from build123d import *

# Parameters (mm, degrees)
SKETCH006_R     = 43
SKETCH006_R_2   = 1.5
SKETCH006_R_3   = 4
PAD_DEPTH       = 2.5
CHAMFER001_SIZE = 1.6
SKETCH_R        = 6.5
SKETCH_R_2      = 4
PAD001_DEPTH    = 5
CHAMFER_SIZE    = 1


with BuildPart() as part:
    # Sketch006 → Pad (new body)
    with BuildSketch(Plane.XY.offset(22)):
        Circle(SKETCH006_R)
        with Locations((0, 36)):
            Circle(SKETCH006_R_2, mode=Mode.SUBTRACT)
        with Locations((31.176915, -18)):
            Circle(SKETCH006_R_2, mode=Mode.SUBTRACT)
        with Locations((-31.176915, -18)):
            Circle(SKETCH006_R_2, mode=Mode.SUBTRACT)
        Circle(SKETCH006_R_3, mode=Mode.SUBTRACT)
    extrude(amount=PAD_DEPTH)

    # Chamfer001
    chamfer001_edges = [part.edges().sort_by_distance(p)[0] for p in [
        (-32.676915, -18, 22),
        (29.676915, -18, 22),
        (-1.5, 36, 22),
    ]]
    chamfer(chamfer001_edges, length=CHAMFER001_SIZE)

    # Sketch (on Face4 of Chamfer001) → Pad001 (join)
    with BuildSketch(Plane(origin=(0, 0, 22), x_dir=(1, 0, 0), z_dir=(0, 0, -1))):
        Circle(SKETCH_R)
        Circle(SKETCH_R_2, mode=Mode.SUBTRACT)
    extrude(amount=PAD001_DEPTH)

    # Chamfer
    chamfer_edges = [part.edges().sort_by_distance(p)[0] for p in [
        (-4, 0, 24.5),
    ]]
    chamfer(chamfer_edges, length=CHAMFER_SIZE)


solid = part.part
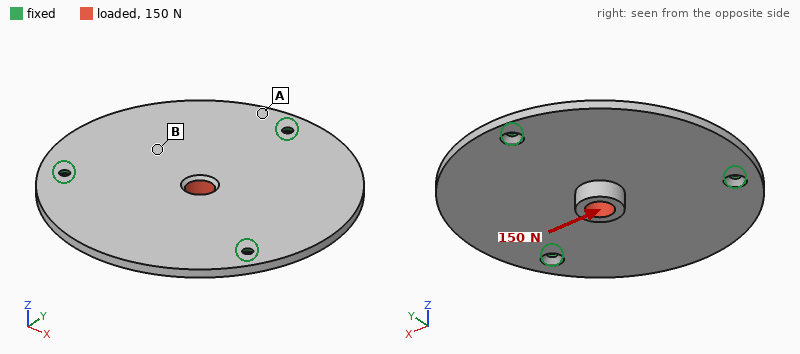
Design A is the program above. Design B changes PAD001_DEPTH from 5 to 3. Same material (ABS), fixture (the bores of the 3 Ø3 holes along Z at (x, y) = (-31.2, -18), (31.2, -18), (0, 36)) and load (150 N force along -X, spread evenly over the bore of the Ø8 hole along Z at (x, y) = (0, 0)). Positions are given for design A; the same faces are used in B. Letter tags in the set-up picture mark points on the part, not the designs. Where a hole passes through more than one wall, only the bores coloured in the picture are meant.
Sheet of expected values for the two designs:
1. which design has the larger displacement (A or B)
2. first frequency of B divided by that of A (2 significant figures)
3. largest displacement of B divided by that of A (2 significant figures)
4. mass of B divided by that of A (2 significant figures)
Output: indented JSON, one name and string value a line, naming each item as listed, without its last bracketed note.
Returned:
{
  "which design has the larger displacement": "A",
  "first frequency of B divided by that of A": "0.99",
  "largest displacement of B divided by that of A": "0.73",
  "mass of B divided by that of A": "0.99"
}
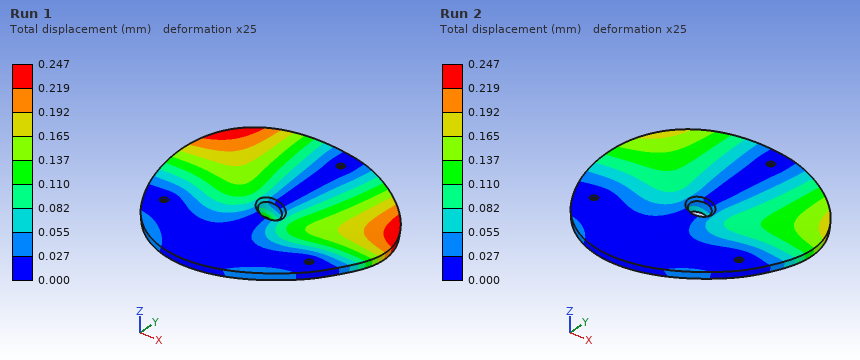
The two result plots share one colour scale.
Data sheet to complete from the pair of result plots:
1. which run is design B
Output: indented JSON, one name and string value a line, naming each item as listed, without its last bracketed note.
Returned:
{
  "which run is design B": "Run 2"
}
